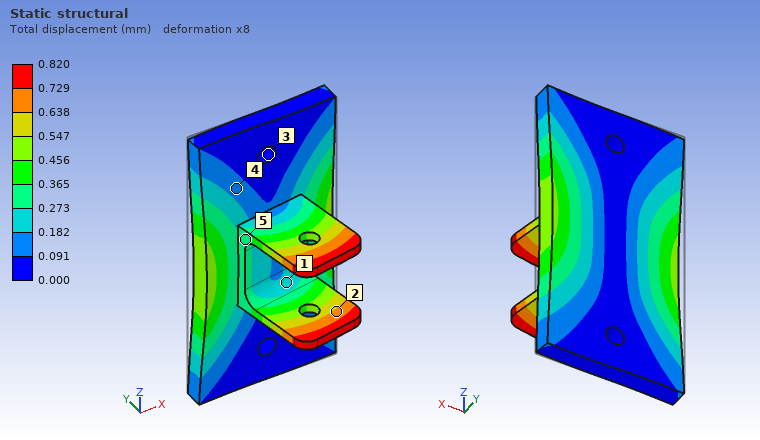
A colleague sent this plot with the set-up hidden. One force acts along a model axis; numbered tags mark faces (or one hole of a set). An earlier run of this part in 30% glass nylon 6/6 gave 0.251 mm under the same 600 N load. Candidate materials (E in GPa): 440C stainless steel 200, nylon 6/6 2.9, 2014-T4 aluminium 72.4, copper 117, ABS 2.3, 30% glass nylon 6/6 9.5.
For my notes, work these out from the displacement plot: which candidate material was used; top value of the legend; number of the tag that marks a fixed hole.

nylon 6/6
0.820 mm
3
